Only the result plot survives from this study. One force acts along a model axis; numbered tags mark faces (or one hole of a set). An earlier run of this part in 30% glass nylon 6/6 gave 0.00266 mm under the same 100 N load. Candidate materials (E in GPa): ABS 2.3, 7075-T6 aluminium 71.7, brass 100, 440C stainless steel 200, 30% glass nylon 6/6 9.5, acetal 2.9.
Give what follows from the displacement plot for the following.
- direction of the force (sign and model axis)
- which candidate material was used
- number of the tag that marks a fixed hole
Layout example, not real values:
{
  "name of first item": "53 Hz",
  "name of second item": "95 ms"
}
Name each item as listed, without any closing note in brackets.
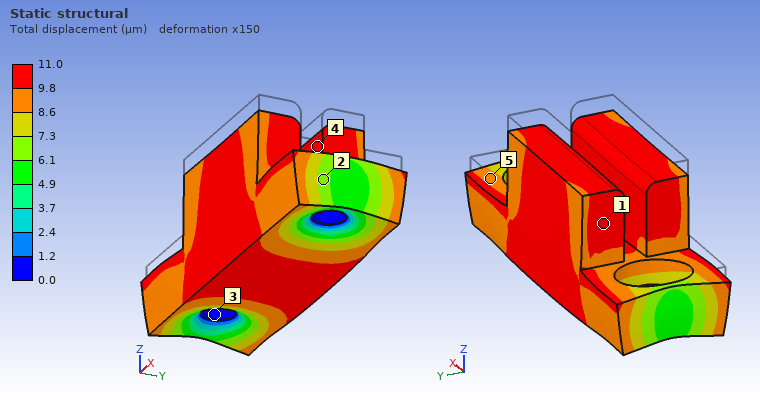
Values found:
{
  "direction of the force": "-Z",
  "which candidate material was used": "ABS",
  "number of the tag that marks a fixed hole": "3"
}
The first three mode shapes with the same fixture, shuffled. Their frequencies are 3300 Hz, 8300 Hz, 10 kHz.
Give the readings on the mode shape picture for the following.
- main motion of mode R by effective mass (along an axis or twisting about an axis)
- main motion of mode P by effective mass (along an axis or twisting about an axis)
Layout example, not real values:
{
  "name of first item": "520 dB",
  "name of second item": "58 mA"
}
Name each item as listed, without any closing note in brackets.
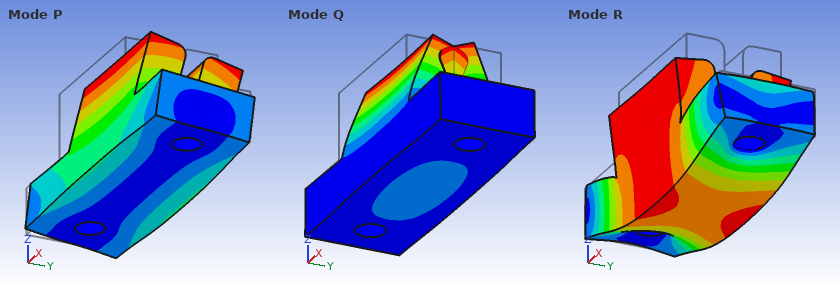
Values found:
{
  "main motion of mode R by effective mass": "along Z",
  "main motion of mode P by effective mass": "along Y"
}
